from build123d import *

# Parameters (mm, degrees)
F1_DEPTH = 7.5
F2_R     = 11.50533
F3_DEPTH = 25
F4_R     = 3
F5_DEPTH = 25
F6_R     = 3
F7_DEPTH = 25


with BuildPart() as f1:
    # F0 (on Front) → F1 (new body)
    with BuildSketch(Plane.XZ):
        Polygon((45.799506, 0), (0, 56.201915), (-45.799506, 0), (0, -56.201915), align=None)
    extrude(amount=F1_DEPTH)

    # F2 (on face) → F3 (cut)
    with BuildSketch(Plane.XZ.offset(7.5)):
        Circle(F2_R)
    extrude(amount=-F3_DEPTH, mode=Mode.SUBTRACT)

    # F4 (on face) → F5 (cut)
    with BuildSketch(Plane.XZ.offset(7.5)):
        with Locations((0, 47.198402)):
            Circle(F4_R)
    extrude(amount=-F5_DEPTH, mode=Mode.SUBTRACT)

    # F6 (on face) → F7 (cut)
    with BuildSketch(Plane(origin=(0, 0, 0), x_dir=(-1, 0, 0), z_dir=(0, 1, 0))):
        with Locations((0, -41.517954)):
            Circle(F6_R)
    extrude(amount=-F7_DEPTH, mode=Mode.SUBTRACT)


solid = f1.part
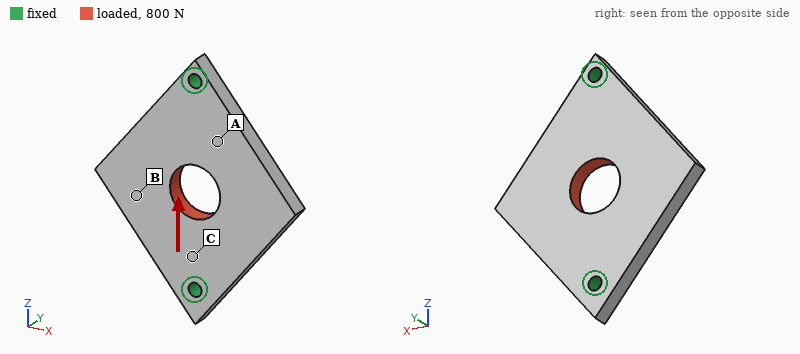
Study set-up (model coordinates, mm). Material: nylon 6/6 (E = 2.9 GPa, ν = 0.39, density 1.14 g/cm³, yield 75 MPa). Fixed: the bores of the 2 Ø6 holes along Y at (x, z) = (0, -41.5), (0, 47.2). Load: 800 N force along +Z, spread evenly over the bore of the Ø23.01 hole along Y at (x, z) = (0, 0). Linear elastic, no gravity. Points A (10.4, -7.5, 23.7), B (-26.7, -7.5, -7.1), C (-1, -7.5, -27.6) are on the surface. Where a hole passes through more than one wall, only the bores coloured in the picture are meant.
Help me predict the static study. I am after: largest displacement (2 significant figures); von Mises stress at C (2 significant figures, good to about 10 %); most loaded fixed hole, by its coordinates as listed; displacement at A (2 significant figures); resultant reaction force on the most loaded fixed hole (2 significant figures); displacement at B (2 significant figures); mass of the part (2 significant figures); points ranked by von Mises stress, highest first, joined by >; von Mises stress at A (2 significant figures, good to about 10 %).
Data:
30 µm
2.6 MPa
(0, -41.5)
20 µm
420 N
20 µm
40 g
C > A > B
1.5 MPa
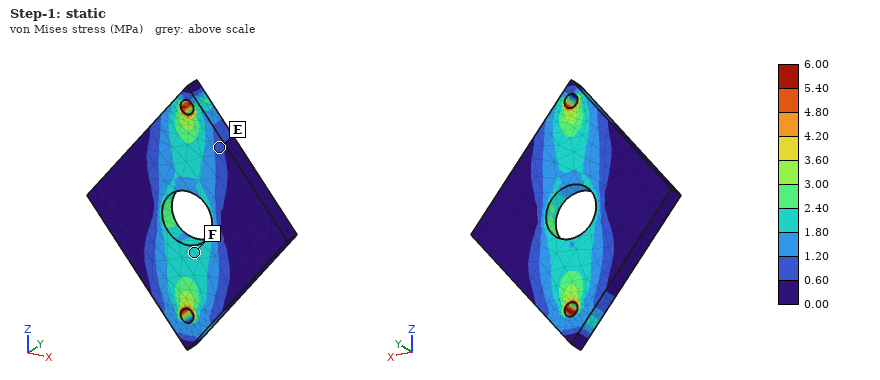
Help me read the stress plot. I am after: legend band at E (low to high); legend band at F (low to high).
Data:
0.60 to 1.20 MPa
1.80 to 2.40 MPa
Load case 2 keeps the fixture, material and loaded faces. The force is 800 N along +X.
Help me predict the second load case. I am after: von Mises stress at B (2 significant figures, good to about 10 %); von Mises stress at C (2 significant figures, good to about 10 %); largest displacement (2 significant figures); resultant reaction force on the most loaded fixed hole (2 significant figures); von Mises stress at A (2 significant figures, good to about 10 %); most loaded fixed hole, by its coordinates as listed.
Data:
1.8 MPa
2.0 MPa
73 µm
420 N
1.5 MPa
(0, -41.5)
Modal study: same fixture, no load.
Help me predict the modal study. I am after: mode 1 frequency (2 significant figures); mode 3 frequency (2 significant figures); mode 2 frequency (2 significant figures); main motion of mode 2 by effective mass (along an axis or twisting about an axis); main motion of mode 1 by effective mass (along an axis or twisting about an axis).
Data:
750 Hz
2500 Hz
940 Hz
along Y
twisting about Z
